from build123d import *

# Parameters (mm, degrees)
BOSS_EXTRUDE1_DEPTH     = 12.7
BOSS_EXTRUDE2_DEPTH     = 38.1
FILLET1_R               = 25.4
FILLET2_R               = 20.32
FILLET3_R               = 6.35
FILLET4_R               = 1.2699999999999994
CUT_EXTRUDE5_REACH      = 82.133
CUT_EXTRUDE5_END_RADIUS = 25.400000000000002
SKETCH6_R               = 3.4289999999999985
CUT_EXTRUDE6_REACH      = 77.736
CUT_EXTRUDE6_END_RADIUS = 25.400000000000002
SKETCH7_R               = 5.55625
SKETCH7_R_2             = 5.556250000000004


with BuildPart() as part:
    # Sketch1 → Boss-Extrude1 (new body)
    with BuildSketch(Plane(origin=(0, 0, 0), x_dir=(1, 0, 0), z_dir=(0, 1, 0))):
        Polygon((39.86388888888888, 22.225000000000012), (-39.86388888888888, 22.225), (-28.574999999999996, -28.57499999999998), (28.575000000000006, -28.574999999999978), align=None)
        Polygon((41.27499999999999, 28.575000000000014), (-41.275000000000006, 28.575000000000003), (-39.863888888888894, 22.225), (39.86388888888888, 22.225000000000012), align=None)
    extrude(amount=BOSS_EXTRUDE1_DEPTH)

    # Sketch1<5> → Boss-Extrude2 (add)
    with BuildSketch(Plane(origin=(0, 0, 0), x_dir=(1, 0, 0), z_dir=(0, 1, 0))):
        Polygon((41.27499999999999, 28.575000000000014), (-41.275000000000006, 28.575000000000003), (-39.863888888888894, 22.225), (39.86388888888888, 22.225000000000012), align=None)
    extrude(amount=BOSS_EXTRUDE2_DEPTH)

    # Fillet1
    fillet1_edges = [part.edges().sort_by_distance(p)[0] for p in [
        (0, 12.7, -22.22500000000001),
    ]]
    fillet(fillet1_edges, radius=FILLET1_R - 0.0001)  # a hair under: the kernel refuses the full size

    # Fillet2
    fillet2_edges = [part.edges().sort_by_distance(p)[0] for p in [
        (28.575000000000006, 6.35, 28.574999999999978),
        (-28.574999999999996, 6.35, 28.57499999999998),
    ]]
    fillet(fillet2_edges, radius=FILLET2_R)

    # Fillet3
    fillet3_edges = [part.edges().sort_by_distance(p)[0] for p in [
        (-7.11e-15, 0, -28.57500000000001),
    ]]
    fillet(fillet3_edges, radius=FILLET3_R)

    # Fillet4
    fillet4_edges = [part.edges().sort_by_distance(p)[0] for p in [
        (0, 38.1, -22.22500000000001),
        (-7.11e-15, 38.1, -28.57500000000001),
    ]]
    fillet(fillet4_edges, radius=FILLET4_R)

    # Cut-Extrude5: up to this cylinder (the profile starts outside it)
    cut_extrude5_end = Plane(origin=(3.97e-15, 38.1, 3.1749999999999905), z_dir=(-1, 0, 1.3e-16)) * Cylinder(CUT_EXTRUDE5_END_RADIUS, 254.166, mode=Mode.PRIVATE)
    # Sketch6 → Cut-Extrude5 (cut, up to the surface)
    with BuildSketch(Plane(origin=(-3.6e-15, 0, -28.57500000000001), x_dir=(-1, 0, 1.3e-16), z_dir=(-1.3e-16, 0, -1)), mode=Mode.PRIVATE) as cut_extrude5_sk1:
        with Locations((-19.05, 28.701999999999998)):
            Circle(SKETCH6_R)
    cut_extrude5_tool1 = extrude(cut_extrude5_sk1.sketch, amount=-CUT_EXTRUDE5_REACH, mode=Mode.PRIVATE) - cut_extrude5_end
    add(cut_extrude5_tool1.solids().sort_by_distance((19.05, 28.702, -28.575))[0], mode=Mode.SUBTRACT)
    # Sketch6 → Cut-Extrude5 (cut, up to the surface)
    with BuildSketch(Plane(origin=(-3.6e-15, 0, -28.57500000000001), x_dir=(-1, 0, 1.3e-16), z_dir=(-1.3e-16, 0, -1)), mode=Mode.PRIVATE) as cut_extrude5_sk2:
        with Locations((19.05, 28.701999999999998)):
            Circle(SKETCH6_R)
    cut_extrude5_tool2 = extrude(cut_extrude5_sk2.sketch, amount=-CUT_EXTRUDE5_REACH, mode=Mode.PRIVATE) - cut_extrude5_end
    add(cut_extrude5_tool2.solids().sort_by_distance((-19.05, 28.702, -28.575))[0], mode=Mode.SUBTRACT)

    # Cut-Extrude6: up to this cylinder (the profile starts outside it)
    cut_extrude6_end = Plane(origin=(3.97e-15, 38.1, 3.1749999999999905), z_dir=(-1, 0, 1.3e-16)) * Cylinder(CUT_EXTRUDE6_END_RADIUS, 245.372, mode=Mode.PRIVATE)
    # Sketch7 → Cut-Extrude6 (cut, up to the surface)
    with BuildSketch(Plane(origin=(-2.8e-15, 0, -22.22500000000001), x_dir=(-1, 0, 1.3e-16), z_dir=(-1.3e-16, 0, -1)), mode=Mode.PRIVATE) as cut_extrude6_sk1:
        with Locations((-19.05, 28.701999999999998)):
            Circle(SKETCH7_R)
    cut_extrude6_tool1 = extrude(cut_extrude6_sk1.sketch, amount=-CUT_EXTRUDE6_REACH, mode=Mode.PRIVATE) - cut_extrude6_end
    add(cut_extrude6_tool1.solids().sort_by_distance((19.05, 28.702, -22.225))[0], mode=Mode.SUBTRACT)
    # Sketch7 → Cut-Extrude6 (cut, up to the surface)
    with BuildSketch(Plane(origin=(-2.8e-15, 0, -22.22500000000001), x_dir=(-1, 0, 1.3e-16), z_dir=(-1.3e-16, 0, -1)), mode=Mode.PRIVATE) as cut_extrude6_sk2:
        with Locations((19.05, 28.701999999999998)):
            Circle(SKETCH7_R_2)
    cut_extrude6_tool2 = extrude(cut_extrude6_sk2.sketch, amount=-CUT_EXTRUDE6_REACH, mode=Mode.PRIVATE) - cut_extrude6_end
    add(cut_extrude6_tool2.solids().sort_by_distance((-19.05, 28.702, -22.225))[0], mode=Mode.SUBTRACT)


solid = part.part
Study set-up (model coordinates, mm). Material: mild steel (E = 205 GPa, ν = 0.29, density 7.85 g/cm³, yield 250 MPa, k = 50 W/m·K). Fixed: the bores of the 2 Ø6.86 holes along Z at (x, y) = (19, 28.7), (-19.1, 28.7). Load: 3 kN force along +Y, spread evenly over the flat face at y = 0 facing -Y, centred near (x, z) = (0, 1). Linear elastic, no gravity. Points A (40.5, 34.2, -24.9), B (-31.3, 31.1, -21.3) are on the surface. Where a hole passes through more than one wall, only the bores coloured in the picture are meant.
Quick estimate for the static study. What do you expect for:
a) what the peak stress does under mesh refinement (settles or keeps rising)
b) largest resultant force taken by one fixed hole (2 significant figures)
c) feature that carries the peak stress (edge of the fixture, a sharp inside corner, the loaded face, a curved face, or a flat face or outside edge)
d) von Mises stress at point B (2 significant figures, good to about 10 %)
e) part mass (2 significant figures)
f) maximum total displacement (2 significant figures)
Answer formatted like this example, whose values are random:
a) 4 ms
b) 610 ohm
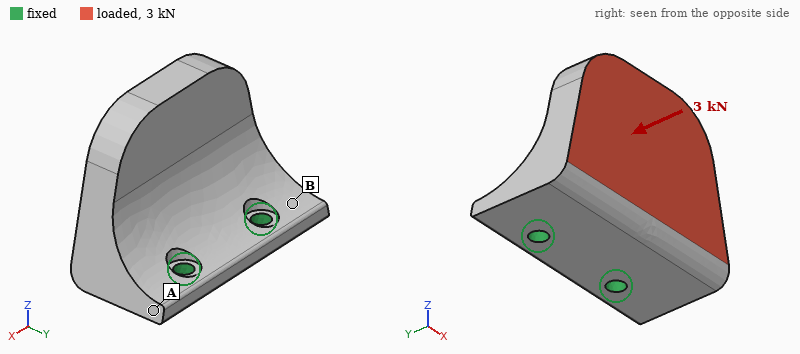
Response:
a) keeps rising
b) 1.5 kN
c) edge of the fixture
d) 50 MPa
e) 560 g
f) 95 µm
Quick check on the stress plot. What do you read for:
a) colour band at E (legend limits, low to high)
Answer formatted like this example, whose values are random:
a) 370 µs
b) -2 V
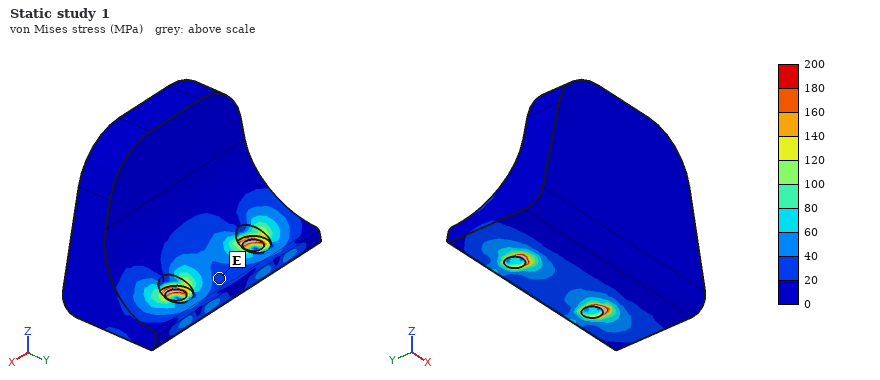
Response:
a) 20 to 40 MPa
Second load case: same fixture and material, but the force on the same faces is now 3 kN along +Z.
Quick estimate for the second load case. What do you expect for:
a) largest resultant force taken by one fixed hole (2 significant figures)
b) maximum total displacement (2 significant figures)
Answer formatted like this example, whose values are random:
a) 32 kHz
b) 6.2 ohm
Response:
a) 1.5 kN
b) 90 µm
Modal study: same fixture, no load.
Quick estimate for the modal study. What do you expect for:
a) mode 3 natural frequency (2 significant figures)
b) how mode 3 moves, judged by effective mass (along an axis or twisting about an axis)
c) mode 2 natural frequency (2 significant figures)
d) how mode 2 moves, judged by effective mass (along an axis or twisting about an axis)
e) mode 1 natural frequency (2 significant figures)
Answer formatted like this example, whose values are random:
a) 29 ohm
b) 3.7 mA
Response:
a) 7600 Hz
b) along X
c) 4300 Hz
d) along X
e) 1700 Hz
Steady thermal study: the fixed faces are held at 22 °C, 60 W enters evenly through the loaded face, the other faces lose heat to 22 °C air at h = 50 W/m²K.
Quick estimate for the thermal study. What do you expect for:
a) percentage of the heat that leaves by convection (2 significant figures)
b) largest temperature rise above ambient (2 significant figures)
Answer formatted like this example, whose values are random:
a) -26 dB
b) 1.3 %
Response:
a) 24 %
b) 48 K
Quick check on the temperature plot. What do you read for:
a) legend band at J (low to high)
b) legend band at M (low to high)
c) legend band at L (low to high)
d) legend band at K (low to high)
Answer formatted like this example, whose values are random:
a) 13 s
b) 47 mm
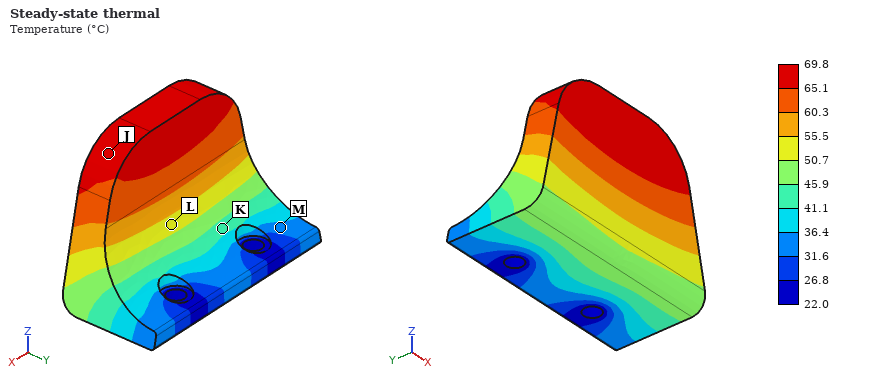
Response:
a) 65.1 to 69.8 °C
b) 31.6 to 36.4 °C
c) 50.7 to 55.5 °C
d) 41.1 to 45.9 °C
